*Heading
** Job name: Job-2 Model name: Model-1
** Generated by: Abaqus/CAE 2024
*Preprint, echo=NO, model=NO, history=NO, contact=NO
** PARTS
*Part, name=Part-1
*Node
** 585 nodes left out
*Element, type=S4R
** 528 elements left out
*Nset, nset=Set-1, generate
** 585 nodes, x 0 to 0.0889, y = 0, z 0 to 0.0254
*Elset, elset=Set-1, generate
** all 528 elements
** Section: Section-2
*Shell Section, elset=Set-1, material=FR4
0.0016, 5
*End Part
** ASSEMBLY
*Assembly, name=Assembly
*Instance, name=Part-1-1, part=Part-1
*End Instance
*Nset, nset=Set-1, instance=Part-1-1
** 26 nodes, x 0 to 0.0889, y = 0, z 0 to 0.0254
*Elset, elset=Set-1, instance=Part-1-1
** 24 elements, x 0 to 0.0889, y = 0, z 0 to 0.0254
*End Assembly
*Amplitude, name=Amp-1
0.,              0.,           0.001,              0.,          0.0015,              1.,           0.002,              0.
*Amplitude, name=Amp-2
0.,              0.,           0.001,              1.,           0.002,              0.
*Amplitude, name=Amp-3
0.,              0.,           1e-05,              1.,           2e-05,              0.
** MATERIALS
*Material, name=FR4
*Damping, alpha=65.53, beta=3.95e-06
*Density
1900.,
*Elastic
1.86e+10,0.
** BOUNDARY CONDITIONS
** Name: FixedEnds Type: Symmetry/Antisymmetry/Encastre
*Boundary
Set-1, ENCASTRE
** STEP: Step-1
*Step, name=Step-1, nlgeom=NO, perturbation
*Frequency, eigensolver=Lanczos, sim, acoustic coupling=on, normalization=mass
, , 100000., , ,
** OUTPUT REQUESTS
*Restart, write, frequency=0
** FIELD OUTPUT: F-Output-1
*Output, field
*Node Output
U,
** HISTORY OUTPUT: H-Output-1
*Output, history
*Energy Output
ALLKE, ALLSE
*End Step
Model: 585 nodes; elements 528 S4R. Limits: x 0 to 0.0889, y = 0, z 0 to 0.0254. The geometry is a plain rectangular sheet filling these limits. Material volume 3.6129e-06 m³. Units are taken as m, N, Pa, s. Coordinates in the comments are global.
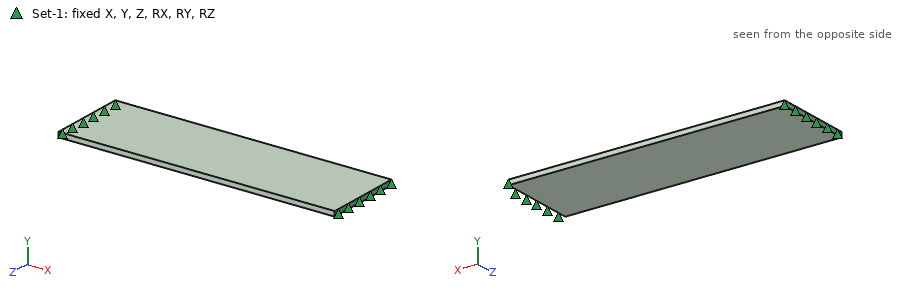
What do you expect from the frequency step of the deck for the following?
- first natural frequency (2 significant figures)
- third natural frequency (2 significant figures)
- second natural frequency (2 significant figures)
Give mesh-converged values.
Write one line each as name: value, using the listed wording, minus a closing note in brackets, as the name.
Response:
first natural frequency: 650 Hz
third natural frequency: 1800 Hz
second natural frequency: 1800 Hz
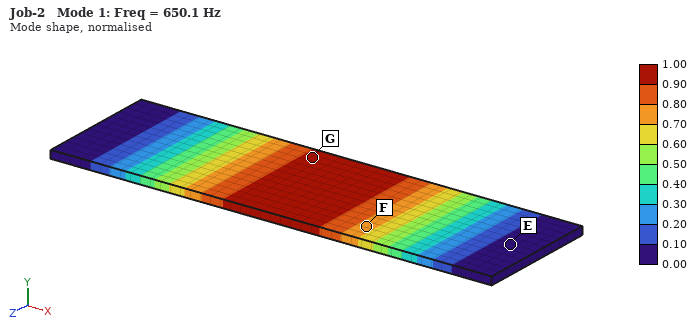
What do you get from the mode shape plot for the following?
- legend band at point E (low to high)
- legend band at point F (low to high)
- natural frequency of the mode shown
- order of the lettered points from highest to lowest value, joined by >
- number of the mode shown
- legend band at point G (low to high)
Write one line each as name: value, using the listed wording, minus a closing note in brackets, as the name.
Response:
legend band at point E: 0.00 to 0.10
legend band at point F: 0.70 to 0.80
natural frequency of the mode shown: 650.1 Hz
order of the lettered points from highest to lowest value, joined by >: G > F > E
number of the mode shown: 1
legend band at point G: 0.90 to 1.00
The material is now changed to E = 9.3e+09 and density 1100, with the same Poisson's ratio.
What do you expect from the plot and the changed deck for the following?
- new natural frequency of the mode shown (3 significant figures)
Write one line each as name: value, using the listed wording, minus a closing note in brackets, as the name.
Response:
new natural frequency of the mode shown: 604 Hz
